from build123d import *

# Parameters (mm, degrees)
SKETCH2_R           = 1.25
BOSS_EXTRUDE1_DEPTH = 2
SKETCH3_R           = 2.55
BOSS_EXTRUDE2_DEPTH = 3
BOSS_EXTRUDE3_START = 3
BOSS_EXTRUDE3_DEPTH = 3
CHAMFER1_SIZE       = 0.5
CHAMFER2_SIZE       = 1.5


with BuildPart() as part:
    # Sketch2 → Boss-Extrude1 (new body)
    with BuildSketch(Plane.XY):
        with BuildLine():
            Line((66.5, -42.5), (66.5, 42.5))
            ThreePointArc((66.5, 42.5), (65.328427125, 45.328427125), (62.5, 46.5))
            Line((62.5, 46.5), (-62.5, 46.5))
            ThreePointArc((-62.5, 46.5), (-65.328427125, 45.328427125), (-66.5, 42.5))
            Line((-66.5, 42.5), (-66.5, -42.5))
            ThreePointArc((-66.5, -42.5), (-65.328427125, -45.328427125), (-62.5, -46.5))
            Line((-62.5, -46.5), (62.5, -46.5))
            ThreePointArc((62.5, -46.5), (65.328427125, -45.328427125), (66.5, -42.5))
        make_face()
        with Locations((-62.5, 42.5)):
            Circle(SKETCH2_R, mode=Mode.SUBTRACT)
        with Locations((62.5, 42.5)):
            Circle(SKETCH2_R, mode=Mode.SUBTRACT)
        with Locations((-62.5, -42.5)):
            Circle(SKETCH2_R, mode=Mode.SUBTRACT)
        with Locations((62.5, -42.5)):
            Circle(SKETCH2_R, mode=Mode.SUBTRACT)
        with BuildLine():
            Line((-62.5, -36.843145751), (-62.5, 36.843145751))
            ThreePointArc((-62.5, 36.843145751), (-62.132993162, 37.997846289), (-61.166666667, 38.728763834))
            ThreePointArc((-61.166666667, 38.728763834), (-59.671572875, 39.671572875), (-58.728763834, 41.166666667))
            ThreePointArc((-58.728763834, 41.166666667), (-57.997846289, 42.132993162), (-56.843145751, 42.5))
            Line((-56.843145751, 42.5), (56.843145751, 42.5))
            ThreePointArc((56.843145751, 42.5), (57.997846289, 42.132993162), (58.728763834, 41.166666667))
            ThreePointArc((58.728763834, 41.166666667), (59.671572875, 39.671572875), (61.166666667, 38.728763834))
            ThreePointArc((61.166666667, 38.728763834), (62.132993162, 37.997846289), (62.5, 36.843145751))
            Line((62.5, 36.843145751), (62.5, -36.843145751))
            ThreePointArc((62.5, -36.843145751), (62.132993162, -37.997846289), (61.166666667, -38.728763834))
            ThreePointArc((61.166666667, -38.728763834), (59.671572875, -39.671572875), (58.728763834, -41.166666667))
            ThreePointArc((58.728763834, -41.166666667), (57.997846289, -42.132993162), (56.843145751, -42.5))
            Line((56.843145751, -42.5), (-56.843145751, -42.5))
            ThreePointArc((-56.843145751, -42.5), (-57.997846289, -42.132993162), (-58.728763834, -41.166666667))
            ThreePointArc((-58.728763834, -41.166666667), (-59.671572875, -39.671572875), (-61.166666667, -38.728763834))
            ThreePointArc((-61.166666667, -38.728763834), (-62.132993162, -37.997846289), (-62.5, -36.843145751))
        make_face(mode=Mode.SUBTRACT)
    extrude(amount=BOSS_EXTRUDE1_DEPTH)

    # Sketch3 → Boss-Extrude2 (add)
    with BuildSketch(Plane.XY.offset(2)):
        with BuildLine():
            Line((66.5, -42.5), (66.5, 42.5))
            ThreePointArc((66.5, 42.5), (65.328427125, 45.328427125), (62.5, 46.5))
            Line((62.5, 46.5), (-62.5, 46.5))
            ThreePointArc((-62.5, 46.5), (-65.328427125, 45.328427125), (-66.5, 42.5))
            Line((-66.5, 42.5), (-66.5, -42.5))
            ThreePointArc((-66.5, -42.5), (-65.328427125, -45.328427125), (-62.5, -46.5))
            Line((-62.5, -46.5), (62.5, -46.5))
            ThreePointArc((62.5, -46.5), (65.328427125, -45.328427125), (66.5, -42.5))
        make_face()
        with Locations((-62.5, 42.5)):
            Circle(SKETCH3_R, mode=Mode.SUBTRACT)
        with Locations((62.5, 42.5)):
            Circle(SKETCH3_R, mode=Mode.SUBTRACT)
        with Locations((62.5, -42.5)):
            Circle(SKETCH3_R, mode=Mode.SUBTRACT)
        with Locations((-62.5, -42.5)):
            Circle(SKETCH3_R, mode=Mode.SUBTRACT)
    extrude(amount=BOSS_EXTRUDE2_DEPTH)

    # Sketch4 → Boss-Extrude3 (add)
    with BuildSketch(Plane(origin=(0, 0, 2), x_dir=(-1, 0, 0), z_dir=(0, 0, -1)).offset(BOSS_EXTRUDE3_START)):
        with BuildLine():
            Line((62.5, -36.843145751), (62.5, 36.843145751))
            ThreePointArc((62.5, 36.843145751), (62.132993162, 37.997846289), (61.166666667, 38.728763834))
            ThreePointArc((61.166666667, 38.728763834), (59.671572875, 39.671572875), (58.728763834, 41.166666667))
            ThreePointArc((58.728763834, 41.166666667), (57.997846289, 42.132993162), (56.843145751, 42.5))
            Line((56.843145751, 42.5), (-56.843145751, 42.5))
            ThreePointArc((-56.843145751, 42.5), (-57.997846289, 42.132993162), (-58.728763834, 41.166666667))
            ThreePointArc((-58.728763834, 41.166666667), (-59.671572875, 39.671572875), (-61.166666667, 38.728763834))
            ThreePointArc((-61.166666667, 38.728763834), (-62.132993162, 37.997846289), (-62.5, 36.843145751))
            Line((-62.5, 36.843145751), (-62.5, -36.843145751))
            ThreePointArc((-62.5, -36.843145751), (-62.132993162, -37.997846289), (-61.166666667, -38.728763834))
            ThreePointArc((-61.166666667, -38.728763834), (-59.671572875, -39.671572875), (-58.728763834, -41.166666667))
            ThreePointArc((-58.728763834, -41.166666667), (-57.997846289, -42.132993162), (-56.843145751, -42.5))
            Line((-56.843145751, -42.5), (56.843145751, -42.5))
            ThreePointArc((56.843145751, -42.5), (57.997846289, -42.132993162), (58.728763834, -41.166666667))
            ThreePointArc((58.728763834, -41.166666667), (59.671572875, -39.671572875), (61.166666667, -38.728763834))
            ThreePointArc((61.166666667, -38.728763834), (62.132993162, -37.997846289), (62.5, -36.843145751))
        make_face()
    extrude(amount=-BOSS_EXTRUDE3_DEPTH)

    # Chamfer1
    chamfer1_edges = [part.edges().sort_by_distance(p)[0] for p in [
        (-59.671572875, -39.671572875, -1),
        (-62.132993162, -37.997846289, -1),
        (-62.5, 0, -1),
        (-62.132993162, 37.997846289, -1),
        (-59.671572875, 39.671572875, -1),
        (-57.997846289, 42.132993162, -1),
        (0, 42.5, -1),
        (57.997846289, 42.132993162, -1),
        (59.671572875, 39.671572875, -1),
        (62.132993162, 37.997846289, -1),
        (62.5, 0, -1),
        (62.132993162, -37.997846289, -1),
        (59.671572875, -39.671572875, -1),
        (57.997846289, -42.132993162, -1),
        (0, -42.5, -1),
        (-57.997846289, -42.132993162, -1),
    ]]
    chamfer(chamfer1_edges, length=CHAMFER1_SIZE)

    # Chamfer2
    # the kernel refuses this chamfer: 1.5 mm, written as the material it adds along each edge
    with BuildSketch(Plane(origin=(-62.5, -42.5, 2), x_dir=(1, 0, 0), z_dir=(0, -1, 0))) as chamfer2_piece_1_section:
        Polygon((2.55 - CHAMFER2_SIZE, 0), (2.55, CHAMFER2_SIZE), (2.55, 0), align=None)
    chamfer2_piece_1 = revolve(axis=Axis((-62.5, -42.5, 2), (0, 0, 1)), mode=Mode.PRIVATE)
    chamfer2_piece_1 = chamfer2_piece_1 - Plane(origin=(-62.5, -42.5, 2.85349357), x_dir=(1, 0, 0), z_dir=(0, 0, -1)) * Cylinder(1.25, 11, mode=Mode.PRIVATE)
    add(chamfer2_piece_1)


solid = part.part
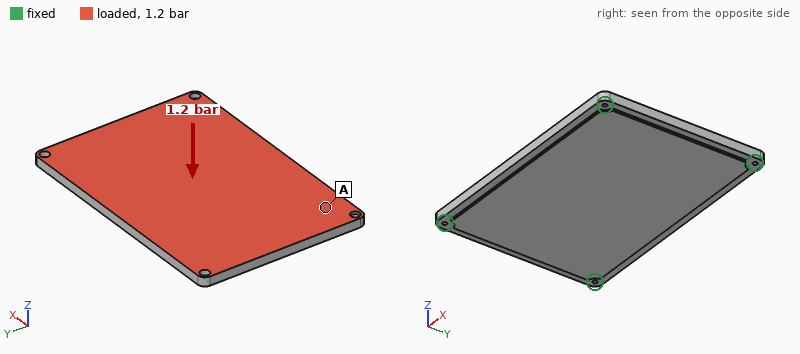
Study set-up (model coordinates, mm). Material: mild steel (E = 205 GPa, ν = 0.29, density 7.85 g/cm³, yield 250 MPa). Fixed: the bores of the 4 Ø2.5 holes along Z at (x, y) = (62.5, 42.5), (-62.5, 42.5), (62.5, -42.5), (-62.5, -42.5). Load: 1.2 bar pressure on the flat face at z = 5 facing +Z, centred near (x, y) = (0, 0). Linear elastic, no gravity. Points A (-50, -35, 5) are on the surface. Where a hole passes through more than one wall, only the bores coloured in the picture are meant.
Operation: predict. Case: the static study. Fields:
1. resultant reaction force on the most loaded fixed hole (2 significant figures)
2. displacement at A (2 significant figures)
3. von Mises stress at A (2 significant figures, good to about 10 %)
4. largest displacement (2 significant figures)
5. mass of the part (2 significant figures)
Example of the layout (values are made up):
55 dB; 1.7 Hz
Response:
710 N; 24 µm; 16 MPa; 78 µm; 570 g
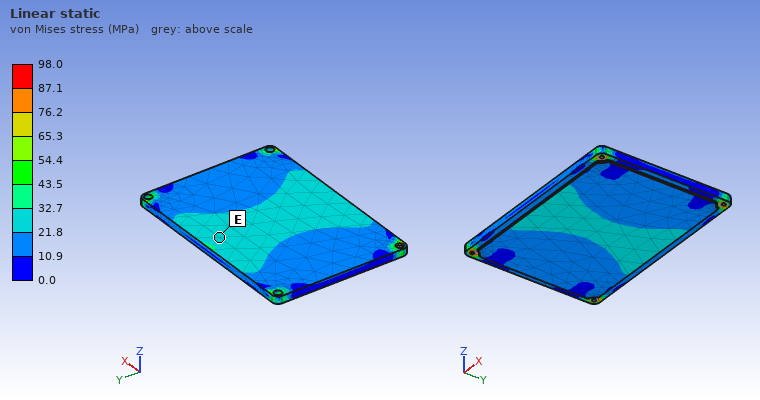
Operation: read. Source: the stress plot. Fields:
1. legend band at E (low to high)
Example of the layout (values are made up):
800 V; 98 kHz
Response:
21.8 to 32.7 MPa
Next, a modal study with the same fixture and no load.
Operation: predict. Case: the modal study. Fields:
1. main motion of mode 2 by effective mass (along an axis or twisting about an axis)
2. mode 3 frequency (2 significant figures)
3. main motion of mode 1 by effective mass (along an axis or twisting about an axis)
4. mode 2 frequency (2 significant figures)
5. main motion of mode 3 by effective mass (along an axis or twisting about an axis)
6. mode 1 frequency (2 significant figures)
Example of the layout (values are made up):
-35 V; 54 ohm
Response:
twisting about X; 2700 Hz; along Z; 2100 Hz; twisting about Y; 1000 Hz
